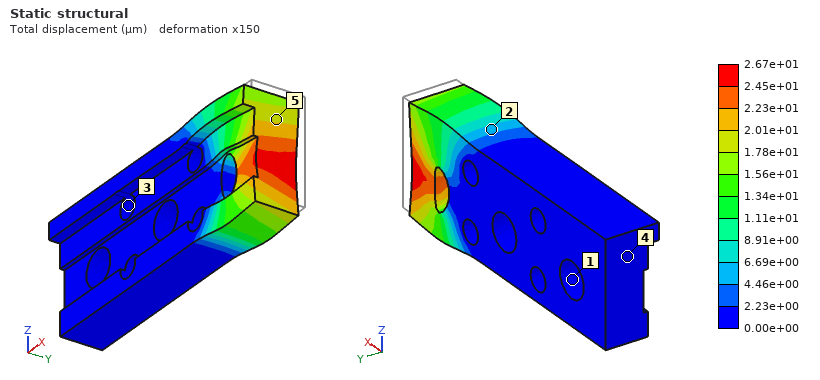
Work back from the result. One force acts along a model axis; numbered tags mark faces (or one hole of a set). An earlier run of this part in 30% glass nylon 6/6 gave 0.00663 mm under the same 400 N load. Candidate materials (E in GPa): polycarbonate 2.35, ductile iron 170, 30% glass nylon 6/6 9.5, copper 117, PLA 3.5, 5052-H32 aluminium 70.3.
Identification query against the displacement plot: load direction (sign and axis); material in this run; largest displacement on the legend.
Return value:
-X
polycarbonate
2.67e+01 µm
